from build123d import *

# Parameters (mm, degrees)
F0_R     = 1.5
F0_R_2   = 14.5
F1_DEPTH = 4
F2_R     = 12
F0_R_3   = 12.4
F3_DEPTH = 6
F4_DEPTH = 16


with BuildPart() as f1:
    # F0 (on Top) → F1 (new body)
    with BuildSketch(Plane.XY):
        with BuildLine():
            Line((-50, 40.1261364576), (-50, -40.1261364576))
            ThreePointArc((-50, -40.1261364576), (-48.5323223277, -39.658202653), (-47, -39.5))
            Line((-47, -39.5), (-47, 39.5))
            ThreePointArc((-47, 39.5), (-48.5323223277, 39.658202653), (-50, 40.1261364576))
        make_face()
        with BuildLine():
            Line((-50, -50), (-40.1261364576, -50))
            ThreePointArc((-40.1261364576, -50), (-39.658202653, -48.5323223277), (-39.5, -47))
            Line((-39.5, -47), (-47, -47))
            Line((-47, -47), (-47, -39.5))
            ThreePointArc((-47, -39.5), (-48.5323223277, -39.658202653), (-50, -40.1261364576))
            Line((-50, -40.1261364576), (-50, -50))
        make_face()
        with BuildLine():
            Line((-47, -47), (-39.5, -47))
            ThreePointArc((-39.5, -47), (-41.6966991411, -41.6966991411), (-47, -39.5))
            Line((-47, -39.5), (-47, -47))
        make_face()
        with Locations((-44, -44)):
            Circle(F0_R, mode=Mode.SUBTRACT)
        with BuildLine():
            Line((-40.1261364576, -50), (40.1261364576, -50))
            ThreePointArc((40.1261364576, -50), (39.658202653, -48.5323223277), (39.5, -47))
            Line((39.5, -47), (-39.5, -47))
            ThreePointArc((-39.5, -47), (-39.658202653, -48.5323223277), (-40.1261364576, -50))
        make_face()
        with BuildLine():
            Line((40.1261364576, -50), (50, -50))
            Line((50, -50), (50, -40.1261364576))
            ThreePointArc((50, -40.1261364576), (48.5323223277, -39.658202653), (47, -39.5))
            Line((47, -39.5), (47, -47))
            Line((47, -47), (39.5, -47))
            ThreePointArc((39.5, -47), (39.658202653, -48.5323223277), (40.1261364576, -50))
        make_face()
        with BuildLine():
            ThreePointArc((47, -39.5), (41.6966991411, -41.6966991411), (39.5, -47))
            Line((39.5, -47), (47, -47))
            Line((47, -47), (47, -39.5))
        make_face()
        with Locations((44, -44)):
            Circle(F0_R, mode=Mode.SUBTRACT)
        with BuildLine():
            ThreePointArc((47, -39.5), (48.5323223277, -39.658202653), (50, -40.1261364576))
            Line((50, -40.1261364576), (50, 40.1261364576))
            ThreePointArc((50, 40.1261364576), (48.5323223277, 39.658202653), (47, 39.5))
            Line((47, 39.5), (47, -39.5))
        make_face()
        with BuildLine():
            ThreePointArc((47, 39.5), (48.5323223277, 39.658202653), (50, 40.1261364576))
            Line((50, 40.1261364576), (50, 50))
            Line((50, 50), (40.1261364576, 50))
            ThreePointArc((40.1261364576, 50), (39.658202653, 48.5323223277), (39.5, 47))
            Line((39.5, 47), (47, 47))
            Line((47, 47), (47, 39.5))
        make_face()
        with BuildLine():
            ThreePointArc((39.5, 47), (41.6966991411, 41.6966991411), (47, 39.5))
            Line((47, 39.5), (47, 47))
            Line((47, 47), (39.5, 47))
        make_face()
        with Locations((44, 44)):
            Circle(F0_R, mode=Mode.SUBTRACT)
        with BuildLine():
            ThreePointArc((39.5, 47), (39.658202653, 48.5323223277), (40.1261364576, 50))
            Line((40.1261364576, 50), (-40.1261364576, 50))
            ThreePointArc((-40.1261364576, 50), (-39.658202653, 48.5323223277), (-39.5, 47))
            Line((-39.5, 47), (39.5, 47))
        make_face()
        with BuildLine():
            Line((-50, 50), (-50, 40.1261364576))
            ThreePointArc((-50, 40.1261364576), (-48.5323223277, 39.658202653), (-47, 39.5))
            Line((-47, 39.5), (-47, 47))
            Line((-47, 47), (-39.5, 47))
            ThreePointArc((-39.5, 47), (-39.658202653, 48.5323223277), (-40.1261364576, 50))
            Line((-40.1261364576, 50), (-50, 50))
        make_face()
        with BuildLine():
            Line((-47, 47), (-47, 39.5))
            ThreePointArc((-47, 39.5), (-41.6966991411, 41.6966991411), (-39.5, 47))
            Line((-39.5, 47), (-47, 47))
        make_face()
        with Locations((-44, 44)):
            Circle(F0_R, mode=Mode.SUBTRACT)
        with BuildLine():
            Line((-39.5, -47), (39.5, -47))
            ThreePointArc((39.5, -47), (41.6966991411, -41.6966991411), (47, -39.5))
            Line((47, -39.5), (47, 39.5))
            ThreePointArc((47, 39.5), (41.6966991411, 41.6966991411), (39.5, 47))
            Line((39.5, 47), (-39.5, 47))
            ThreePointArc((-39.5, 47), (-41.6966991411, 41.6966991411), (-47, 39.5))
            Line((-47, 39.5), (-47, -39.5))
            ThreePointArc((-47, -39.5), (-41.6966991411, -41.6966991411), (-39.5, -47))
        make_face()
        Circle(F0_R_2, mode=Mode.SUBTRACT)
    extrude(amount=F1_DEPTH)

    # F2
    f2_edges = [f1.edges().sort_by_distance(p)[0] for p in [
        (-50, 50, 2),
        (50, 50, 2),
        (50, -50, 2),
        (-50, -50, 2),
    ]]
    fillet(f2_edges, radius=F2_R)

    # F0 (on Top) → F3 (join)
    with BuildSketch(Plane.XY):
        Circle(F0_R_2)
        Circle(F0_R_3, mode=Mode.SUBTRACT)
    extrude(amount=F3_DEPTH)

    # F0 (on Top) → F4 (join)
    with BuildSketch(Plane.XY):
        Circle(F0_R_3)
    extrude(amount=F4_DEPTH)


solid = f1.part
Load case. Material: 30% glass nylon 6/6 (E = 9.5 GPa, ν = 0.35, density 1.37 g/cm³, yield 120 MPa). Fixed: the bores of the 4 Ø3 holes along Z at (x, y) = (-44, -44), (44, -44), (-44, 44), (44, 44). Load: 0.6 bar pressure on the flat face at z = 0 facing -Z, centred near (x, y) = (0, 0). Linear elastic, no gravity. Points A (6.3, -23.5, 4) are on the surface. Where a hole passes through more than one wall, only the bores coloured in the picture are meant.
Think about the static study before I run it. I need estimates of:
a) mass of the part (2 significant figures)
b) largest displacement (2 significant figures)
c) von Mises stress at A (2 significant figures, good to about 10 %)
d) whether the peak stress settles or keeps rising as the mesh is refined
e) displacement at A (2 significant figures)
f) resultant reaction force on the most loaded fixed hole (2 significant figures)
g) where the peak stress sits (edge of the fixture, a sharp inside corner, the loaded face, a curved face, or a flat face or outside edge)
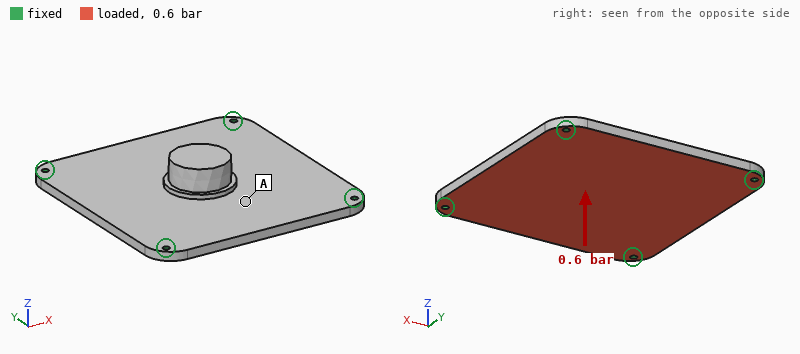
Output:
62 g
0.47 mm
9.2 MPa
keeps rising
0.43 mm
150 N
edge of the fixture
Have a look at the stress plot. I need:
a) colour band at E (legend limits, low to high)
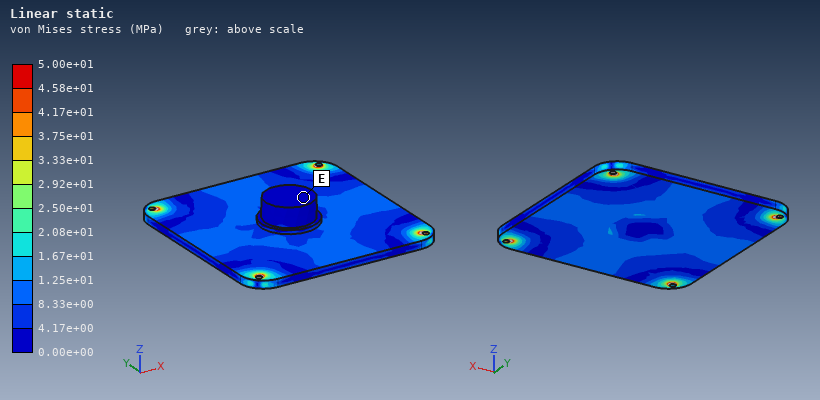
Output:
0.00e+00 to 4.17e+00 MPa
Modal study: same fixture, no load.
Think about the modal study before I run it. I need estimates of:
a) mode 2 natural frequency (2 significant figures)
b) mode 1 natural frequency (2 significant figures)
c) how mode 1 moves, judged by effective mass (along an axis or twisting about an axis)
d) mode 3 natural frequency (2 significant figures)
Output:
1400 Hz
750 Hz
along Z
1400 Hz
